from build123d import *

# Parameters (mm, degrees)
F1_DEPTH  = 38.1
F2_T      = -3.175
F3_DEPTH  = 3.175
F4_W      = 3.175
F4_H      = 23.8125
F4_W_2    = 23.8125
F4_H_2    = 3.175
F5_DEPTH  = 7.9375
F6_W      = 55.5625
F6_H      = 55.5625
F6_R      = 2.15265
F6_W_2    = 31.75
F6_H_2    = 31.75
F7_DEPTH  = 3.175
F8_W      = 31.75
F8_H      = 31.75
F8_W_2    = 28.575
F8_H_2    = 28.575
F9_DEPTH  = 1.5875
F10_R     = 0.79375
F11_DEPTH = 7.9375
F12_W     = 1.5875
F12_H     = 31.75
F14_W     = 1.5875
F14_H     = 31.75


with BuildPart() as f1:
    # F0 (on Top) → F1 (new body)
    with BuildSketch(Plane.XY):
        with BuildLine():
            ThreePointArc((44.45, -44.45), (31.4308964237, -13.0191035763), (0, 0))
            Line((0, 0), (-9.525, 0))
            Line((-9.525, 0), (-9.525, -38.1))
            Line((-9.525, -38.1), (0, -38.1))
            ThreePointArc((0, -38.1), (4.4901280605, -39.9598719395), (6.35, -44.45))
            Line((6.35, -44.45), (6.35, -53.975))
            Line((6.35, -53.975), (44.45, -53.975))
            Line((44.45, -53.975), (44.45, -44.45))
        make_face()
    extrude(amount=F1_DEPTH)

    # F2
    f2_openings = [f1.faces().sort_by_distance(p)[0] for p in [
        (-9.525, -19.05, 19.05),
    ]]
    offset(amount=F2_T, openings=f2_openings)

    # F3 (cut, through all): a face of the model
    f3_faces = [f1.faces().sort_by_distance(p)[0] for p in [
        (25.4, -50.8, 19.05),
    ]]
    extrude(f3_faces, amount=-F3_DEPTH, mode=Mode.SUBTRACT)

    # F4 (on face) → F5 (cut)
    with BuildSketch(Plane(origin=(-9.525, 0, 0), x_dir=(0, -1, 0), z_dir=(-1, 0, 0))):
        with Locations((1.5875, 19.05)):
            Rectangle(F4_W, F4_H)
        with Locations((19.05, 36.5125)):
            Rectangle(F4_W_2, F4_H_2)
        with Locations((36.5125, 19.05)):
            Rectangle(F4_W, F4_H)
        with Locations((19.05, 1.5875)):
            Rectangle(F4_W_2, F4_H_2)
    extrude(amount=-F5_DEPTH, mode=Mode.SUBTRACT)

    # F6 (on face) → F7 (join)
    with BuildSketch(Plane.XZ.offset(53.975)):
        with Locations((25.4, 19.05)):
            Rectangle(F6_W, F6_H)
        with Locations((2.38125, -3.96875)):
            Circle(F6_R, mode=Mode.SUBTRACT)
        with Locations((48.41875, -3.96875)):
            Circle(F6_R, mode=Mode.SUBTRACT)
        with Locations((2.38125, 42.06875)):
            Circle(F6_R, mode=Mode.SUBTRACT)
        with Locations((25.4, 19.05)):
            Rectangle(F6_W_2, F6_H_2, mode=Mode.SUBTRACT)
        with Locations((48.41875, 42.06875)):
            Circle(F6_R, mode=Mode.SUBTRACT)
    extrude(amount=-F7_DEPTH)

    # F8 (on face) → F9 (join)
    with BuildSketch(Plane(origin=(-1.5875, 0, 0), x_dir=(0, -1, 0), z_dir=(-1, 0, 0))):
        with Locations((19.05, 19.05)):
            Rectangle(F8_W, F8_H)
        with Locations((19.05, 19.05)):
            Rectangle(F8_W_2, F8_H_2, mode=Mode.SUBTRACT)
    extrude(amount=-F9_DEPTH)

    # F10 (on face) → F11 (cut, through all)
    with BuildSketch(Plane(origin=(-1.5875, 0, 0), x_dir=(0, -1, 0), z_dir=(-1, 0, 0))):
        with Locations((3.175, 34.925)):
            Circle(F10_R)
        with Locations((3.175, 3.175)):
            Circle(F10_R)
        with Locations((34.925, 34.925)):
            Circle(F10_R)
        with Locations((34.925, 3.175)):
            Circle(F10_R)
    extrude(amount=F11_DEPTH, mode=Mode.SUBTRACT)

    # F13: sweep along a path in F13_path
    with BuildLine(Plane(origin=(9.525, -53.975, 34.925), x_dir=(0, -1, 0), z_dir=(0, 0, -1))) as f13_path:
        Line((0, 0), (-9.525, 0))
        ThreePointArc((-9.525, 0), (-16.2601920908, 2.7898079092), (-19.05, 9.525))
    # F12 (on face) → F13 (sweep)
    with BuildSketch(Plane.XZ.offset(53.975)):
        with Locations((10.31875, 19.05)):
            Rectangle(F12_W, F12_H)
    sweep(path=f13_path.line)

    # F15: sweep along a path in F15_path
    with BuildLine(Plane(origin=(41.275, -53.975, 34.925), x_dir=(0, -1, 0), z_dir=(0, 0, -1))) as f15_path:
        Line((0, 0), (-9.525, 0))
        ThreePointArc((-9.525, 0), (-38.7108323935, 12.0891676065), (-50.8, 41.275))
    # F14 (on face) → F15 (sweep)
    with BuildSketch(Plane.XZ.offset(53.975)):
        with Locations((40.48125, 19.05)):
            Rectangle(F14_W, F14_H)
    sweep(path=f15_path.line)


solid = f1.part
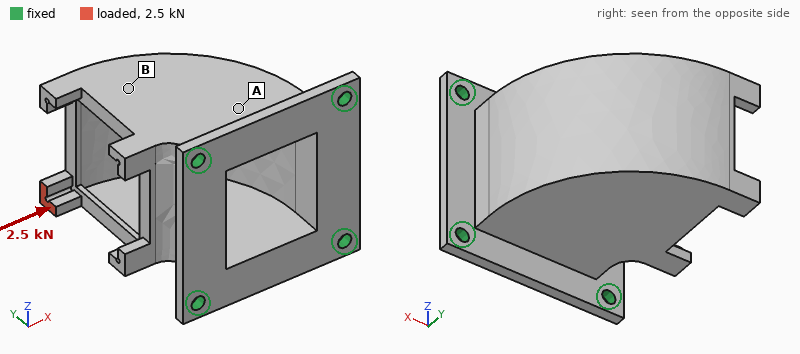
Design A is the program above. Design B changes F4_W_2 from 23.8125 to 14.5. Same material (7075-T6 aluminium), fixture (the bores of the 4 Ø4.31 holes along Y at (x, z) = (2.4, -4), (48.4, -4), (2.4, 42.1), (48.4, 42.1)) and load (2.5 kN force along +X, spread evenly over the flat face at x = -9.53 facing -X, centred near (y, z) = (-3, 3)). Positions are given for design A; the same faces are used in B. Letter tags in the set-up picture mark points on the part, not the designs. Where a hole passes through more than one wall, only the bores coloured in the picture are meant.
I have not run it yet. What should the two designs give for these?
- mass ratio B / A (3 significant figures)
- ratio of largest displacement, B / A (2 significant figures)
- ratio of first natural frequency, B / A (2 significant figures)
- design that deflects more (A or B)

1.01
0.91
0.99
A
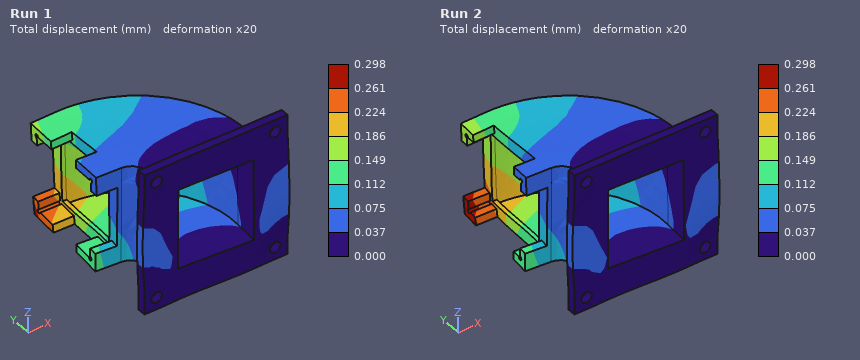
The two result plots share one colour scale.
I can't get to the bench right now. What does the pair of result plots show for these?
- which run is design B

Run 1
